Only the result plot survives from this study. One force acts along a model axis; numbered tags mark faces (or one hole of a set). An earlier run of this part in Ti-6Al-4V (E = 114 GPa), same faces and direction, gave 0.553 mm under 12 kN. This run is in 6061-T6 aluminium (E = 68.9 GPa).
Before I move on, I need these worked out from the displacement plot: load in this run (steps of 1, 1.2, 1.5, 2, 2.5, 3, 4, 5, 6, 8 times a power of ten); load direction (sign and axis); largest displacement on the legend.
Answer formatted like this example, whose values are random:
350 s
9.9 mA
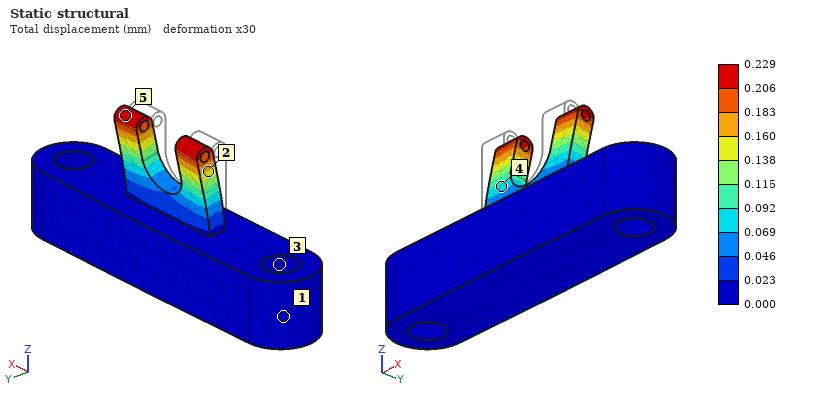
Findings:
3 kN
+Y
0.229 mm
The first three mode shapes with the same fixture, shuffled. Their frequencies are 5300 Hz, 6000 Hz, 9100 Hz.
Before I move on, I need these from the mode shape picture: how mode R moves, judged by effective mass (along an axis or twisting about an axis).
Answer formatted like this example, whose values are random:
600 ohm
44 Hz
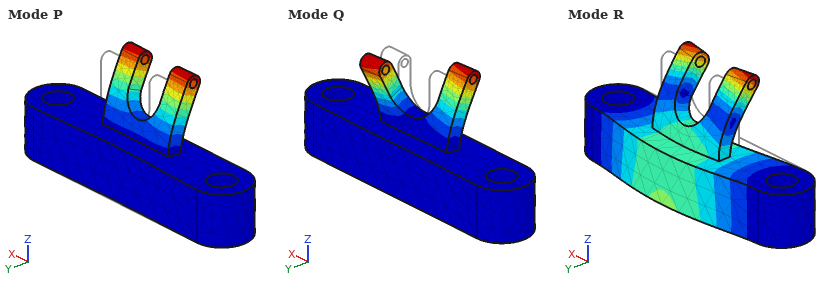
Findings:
along Y
